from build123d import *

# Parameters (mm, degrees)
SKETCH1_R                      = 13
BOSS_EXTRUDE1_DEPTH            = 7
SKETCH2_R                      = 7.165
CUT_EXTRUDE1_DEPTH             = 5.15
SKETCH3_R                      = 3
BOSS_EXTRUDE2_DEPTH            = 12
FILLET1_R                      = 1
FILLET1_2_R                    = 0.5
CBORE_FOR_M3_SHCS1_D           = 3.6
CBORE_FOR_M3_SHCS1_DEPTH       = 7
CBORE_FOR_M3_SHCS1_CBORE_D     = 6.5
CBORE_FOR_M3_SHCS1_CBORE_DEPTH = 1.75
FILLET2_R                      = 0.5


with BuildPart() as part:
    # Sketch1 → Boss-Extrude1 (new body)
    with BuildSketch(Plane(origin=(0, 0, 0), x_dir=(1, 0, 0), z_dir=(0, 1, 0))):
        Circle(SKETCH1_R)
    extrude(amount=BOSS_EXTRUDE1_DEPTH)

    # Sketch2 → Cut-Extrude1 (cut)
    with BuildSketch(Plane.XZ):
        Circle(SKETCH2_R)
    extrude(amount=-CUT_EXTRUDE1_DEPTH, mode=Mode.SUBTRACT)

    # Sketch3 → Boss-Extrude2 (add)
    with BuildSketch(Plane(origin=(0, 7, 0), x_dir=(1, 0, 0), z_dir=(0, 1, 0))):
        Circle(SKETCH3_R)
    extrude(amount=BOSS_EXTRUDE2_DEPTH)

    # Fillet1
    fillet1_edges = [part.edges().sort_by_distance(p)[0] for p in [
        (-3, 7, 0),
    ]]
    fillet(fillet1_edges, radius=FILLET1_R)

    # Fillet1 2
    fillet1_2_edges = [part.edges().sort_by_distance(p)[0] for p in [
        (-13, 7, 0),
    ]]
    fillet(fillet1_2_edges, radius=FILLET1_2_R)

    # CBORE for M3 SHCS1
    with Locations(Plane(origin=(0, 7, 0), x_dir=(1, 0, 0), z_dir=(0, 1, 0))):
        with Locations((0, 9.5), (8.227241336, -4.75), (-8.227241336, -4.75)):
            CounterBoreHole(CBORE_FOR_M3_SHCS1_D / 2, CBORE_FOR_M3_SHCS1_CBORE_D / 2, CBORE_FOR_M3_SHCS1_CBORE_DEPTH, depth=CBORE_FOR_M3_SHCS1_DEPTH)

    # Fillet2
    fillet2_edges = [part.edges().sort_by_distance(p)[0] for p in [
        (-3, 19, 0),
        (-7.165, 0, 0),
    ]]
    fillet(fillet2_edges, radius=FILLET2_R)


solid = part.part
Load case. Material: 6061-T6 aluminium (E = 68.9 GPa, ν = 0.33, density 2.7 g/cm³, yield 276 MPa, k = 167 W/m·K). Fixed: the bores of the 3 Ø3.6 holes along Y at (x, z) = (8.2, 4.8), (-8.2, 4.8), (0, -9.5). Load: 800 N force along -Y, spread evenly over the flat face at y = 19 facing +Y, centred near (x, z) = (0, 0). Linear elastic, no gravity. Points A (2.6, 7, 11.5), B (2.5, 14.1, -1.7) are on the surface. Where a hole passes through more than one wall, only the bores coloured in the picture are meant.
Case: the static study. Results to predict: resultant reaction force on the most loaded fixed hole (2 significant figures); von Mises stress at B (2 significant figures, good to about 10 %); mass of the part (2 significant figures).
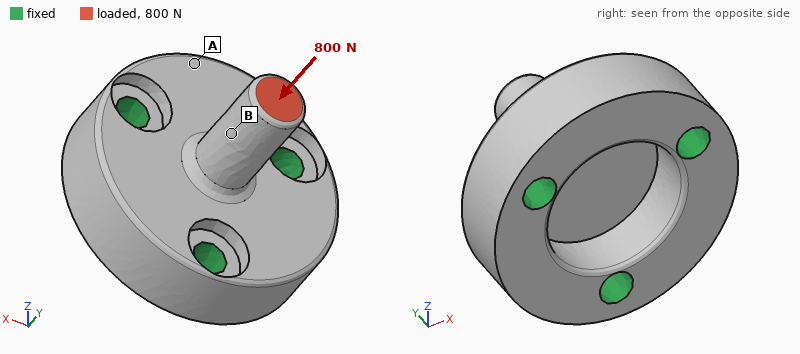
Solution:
310 N
28 MPa
7.8 g
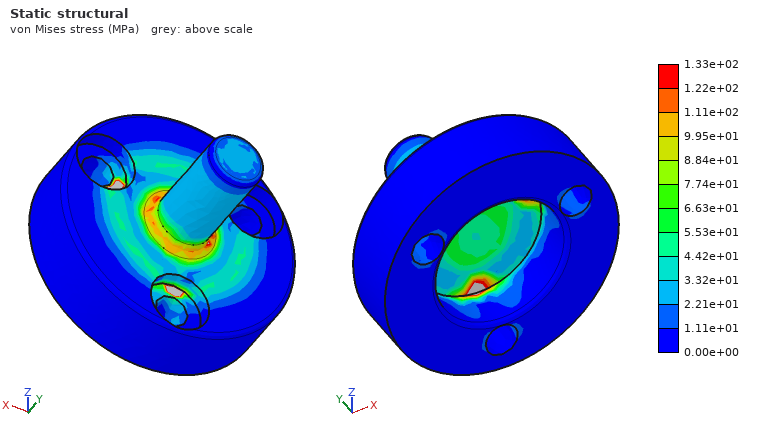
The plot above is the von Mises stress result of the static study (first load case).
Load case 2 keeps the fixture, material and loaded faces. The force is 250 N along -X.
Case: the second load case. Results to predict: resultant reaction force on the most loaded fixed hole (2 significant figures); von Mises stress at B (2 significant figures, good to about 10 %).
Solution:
240 N
51 MPa
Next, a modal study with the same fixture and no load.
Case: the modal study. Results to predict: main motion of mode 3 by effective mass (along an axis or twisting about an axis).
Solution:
along Y
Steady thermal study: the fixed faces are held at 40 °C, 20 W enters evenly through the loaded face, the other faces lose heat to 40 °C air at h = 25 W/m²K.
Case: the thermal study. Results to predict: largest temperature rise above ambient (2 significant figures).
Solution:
69 K
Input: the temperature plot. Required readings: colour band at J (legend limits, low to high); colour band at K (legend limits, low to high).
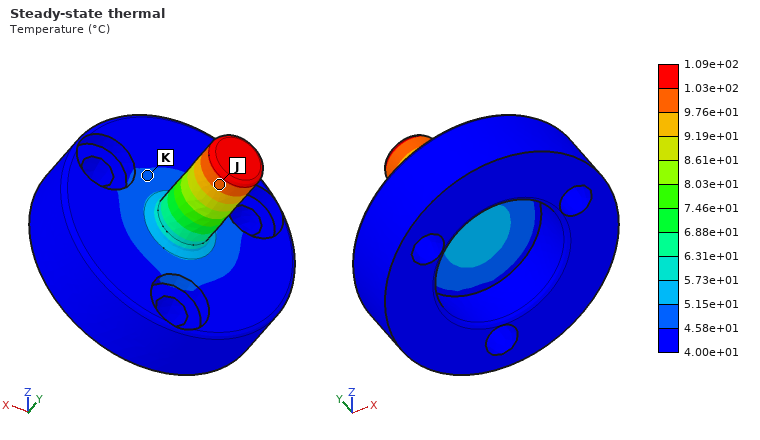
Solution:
9.76e+01 to 1.03e+02 °C
4.58e+01 to 5.15e+01 °C
